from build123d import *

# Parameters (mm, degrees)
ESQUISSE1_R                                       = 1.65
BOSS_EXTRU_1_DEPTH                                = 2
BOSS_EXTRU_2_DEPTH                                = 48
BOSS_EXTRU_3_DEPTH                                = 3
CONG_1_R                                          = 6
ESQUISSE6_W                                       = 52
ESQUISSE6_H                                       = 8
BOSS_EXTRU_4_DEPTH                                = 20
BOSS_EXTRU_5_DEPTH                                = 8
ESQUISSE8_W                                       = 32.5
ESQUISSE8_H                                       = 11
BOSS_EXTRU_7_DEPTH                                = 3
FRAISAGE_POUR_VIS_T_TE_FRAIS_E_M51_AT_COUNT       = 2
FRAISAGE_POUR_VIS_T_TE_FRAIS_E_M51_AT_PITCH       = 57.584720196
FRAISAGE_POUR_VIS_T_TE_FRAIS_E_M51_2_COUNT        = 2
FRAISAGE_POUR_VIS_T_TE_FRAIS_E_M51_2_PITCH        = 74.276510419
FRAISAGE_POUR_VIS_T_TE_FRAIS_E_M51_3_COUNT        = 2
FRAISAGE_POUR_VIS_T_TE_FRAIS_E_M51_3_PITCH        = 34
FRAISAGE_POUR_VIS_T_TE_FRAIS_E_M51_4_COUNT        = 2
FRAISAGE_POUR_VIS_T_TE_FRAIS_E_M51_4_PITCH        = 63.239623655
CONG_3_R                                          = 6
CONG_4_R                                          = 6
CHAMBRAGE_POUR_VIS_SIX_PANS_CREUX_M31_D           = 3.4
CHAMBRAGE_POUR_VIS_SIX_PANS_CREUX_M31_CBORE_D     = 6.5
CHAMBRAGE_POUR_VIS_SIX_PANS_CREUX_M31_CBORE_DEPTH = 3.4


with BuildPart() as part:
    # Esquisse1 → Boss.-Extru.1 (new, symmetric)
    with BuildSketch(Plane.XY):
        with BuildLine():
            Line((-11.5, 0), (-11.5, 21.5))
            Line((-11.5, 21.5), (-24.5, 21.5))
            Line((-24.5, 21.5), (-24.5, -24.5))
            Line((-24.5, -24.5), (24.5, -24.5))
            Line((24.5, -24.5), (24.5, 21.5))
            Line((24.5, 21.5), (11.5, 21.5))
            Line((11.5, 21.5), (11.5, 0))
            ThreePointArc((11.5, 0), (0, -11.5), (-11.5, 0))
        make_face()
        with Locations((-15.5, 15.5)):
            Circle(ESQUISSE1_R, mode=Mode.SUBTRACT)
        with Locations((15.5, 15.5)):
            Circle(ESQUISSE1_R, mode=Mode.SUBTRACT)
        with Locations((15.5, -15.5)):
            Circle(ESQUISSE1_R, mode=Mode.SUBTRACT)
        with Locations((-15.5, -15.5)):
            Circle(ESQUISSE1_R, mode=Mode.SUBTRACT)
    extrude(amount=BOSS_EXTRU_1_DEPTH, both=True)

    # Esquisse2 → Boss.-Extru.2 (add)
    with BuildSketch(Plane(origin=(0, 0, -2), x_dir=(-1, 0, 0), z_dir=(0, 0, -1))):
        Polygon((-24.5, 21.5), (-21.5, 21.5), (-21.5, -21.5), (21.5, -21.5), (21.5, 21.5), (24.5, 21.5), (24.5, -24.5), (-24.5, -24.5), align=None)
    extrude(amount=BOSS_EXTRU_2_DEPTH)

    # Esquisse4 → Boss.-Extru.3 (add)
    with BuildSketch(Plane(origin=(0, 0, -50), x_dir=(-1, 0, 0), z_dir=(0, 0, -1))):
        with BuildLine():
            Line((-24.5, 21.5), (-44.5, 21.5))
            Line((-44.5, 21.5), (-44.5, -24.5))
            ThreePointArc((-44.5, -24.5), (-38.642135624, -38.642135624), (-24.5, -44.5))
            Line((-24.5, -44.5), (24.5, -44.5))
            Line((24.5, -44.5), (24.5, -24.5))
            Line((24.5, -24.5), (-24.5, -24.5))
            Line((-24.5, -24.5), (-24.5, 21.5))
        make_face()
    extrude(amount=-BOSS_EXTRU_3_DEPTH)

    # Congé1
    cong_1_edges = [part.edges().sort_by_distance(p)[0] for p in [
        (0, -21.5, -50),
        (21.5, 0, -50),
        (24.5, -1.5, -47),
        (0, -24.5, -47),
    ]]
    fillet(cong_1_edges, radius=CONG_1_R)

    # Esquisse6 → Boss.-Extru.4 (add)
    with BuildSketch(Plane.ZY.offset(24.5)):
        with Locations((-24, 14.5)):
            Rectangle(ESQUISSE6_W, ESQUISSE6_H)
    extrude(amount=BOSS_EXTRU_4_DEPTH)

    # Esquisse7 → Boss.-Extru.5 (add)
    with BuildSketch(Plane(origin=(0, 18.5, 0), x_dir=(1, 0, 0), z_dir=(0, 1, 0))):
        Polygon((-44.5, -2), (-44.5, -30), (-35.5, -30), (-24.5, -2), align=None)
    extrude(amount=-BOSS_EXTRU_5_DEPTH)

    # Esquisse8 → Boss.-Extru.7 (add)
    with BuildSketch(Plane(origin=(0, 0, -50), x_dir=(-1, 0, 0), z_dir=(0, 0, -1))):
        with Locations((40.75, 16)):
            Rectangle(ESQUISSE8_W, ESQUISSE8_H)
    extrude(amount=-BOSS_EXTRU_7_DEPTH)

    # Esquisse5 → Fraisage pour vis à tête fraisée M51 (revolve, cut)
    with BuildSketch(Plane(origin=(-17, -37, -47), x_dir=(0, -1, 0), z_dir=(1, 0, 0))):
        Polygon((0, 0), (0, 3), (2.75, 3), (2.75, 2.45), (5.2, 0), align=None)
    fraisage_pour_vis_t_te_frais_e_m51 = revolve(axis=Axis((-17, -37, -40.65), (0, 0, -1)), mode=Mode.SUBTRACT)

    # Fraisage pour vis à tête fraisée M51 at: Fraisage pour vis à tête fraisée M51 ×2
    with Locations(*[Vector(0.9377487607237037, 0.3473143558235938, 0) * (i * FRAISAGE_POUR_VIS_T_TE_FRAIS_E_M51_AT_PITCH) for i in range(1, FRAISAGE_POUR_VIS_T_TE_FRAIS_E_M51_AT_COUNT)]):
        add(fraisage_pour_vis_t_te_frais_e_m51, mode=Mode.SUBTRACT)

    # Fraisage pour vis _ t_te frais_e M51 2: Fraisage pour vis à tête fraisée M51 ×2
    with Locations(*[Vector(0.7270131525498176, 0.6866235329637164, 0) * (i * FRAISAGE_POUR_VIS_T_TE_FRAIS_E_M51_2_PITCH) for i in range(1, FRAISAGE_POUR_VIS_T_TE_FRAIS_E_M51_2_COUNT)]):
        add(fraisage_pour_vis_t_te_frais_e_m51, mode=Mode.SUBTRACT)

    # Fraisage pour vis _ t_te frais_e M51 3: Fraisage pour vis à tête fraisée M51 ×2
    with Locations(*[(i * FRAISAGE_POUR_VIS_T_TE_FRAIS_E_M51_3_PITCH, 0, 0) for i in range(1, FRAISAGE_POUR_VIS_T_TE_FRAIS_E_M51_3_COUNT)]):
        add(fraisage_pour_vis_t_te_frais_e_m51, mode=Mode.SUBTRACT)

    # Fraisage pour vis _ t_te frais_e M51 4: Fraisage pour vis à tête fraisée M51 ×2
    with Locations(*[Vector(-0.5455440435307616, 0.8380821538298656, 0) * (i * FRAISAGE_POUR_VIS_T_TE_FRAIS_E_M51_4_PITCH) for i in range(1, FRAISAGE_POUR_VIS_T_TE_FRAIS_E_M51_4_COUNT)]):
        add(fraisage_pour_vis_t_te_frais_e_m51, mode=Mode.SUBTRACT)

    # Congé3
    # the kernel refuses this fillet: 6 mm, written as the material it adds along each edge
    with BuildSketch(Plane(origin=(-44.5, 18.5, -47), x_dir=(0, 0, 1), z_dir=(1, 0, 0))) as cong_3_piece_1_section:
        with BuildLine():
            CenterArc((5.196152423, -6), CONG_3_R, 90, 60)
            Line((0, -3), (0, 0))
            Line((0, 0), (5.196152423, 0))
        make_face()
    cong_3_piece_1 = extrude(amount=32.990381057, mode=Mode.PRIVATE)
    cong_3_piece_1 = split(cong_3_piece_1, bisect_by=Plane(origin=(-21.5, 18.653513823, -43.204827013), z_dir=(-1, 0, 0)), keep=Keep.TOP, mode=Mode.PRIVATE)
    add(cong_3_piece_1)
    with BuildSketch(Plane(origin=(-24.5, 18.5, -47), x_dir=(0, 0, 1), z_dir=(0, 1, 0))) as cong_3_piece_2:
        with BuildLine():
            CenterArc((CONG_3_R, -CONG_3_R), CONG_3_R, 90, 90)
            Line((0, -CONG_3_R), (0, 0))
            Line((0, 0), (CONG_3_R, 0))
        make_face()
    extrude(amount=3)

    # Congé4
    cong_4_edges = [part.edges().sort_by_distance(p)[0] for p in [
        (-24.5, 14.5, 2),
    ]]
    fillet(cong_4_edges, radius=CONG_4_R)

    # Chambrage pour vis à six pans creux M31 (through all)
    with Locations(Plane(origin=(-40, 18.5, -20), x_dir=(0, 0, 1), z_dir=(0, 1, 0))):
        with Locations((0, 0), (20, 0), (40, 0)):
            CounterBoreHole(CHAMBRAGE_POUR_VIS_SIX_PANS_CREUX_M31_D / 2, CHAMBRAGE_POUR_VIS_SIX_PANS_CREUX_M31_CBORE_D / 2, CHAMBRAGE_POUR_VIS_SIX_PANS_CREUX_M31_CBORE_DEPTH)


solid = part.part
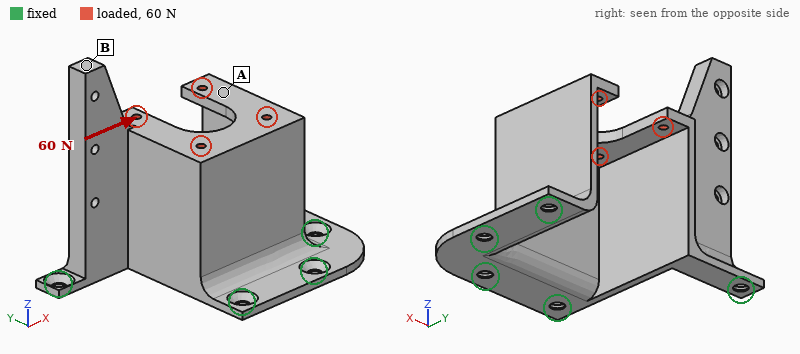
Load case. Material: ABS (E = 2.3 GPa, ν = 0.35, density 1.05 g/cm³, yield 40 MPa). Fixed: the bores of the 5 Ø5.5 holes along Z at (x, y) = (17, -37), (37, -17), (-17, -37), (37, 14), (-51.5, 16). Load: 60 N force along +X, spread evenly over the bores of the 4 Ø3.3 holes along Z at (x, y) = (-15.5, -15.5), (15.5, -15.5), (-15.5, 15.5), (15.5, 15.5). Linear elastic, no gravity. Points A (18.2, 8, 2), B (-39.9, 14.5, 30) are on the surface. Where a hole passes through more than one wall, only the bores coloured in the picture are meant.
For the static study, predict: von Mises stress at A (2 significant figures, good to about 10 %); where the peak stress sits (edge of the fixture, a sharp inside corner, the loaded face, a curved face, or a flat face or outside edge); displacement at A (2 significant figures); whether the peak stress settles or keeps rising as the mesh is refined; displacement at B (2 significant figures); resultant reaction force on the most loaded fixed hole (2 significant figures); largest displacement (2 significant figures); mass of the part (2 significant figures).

2.4 MPa
edge of the fixture
0.71 mm
keeps rising
1.5 mm
50 N
1.5 mm
46 g
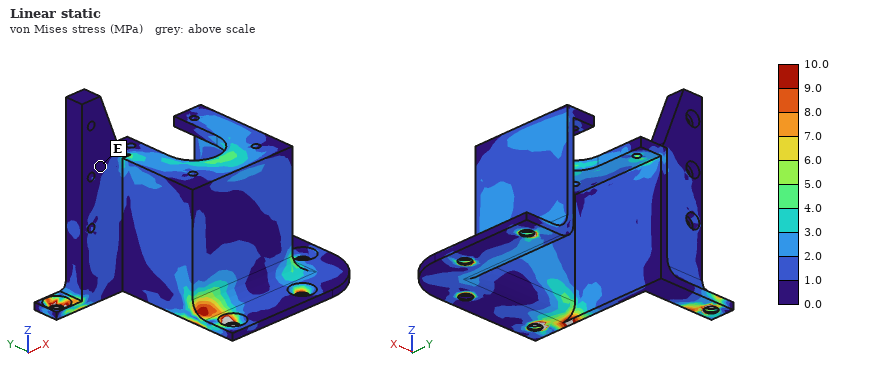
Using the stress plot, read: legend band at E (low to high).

0.0 to 1.0 MPa
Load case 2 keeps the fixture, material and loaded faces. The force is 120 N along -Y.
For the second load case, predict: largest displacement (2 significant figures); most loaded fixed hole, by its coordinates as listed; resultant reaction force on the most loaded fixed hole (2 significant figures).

1.3 mm
(-17, -37)
120 N
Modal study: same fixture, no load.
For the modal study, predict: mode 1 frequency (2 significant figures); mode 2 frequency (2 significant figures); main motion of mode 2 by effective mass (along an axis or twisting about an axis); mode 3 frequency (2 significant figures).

240 Hz
580 Hz
along Y
870 Hz
